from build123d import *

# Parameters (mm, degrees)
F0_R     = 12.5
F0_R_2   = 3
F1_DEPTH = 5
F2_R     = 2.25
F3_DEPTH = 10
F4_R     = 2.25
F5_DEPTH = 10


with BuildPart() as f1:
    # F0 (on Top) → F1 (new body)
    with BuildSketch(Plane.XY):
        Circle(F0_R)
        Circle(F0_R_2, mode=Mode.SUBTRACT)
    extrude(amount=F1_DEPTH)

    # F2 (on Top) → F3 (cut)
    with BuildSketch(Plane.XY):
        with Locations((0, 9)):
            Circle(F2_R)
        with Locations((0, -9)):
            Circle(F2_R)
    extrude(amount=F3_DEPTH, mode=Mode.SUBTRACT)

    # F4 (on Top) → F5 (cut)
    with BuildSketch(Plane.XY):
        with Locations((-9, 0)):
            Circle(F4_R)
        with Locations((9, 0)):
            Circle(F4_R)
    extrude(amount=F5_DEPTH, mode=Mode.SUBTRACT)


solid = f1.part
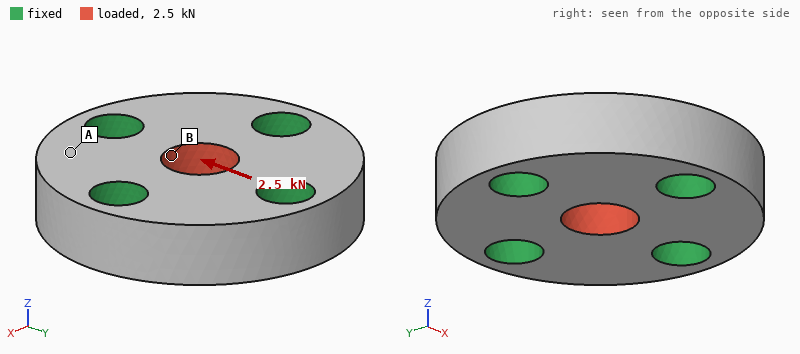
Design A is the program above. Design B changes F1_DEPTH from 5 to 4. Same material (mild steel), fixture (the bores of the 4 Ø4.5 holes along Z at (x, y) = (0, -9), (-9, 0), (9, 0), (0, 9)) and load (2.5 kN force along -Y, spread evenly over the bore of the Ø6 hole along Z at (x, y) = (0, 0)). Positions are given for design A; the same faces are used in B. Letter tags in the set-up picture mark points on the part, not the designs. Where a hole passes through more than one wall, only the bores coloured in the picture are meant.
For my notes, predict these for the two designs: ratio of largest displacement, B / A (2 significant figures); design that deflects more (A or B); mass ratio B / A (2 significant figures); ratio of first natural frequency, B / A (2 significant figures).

1.3
B
0.80
0.91
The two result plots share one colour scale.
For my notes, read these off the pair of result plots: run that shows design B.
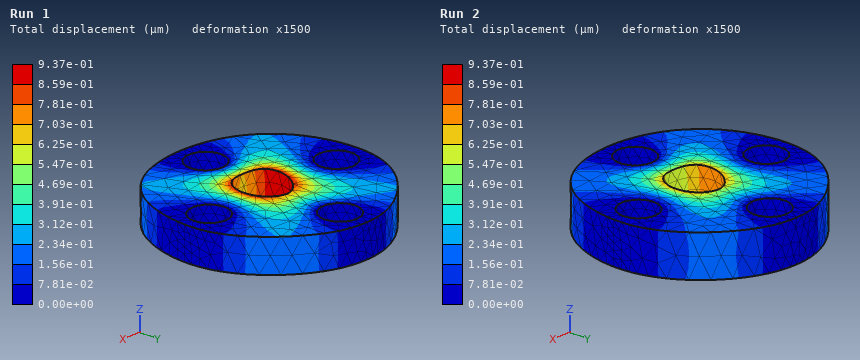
Run 1
